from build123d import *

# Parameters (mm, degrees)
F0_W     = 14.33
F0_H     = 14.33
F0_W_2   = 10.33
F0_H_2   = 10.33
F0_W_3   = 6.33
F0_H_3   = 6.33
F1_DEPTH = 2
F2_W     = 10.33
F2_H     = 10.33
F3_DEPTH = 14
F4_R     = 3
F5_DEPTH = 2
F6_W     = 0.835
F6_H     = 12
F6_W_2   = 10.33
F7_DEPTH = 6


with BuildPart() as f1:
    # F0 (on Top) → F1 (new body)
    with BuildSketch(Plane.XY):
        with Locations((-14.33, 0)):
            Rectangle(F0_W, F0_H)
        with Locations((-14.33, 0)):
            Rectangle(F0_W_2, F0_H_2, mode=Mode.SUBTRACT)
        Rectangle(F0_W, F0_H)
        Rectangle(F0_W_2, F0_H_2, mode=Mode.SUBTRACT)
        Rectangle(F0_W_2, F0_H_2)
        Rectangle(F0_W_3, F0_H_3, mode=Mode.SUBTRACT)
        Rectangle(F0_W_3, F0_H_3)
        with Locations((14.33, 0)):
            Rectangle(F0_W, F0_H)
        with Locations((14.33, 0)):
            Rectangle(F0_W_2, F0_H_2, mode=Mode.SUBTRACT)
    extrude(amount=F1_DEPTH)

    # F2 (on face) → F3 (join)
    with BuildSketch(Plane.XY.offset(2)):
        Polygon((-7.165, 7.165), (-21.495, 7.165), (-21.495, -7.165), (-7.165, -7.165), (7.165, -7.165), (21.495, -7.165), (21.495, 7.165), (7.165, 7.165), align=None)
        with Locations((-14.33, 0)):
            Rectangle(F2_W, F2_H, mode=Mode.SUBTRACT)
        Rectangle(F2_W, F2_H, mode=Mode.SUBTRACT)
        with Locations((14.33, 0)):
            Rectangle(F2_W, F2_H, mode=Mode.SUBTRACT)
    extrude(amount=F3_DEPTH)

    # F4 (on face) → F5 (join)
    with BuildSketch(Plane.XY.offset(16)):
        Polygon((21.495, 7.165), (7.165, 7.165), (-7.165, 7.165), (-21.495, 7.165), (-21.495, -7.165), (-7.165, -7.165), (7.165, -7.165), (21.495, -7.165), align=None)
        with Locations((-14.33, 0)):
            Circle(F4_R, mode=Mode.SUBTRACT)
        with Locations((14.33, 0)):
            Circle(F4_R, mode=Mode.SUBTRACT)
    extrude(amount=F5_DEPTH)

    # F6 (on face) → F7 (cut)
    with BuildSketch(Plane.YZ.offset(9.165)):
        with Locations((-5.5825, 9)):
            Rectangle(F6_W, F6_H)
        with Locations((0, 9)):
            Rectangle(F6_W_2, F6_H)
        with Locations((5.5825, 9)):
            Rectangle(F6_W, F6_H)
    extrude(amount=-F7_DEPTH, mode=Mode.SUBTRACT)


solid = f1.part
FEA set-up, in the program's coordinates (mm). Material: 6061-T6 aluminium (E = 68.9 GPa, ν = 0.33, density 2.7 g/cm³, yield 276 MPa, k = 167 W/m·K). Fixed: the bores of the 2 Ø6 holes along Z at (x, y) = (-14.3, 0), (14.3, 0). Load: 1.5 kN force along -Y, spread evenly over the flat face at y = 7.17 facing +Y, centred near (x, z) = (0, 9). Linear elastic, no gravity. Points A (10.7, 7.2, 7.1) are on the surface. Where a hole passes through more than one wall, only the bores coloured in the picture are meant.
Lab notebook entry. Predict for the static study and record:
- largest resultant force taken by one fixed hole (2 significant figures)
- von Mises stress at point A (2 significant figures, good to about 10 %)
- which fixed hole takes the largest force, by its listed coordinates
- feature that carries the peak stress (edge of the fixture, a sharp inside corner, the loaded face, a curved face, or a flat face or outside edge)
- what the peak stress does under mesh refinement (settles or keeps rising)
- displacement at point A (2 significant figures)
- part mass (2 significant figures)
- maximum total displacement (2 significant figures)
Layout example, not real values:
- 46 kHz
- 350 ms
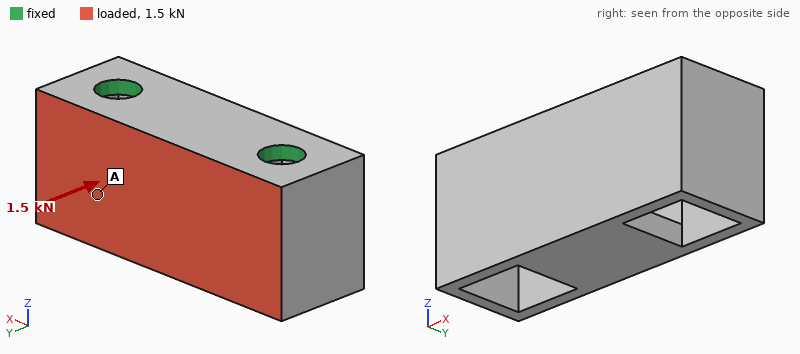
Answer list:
- 810 N
- 29 MPa
- (-14.3, 0)
- edge of the fixture
- keeps rising
- 60 µm
- 15 g
- 80 µm
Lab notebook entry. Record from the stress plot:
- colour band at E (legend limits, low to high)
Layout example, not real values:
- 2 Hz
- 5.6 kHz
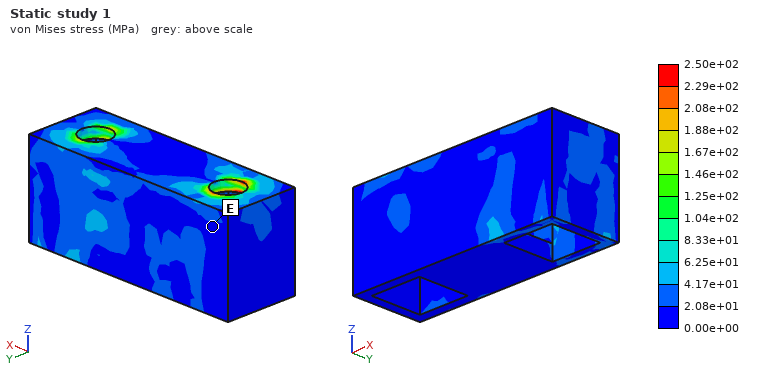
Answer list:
- 0.00e+00 to 2.08e+01 MPa
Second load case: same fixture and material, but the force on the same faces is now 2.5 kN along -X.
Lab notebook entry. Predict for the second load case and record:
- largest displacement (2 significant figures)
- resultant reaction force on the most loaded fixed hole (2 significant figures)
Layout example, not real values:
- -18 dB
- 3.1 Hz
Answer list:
- 25 µm
- 1.5 kN
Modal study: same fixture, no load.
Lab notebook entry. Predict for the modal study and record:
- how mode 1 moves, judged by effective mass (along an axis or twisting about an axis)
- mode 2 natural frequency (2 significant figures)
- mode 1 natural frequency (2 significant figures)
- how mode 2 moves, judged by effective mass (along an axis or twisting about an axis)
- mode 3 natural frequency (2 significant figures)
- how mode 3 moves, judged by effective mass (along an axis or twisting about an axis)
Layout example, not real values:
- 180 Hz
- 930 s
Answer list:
- along Y
- 16 kHz
- 6900 Hz
- twisting about Z
- 17 kHz
- along X
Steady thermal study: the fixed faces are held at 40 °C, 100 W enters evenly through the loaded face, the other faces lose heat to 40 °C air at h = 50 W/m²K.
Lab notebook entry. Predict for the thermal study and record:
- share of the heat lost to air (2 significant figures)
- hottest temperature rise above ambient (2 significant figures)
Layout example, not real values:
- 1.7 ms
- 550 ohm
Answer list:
- 6.3 %
- 53 K
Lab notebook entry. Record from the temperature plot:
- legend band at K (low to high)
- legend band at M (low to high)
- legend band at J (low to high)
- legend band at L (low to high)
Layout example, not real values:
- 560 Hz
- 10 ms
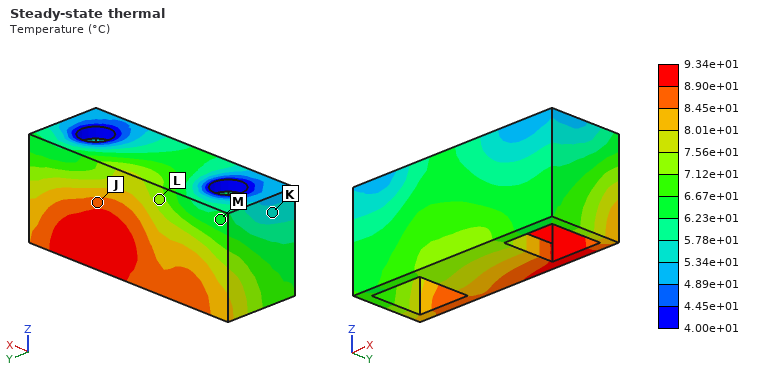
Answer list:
- 5.34e+01 to 5.78e+01 °C
- 6.23e+01 to 6.67e+01 °C
- 8.45e+01 to 8.90e+01 °C
- 7.12e+01 to 7.56e+01 °C
